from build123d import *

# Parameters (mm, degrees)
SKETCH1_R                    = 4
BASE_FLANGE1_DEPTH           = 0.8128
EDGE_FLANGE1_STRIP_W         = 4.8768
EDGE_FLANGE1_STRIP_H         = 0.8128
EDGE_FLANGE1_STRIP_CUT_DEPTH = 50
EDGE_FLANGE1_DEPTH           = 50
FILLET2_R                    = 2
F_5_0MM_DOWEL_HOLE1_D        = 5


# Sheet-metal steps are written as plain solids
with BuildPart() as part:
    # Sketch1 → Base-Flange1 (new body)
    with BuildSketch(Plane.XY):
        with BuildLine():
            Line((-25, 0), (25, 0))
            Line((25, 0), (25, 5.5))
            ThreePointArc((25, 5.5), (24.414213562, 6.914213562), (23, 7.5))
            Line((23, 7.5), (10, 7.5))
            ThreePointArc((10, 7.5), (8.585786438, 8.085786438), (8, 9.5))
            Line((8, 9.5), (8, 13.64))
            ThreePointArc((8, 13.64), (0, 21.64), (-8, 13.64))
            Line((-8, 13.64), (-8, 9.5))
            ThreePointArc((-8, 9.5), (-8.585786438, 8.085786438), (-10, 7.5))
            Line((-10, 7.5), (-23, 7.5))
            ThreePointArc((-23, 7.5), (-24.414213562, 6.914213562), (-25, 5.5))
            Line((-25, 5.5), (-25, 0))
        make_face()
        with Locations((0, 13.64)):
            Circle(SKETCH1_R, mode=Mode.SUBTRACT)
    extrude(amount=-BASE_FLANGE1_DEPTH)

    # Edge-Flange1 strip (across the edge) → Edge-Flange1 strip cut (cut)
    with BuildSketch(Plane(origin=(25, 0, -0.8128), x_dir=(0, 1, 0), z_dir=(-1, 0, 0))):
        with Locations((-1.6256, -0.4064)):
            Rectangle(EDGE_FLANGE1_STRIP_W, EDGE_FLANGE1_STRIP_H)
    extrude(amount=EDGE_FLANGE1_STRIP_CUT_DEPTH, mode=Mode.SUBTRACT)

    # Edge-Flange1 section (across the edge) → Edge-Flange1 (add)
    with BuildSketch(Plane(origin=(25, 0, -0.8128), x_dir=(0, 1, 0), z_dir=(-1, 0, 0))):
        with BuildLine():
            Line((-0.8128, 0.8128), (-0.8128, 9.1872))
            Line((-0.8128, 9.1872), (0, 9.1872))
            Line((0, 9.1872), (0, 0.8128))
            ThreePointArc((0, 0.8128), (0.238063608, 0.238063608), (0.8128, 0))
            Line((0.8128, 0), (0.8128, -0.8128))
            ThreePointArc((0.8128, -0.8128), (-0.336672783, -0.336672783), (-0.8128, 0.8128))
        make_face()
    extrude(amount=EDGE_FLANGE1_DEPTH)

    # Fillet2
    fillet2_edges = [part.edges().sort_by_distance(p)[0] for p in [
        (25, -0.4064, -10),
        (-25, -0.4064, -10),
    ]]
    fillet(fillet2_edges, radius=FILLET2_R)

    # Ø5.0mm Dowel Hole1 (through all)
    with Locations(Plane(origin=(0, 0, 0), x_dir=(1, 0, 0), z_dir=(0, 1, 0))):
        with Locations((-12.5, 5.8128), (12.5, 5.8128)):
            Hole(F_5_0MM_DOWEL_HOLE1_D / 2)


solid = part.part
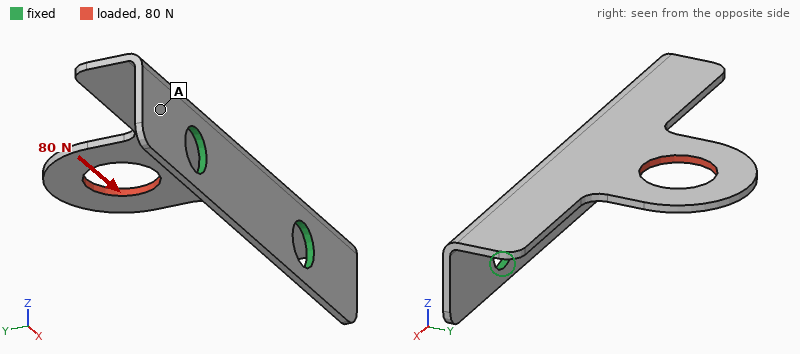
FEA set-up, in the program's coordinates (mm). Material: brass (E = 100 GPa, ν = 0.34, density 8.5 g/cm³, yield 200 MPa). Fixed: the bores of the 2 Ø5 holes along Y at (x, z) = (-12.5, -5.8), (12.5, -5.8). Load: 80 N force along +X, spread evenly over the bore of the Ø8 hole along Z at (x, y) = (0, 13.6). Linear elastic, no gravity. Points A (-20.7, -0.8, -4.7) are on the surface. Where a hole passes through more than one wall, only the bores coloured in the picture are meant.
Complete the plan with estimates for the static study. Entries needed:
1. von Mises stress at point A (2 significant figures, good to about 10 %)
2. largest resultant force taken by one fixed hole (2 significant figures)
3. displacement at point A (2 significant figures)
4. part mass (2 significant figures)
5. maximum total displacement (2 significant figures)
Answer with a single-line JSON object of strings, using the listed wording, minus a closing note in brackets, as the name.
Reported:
{"von Mises stress at point A": "12 MPa", "largest resultant force taken by one fixed hole": "59 N", "displacement at point A": "4.6 µm", "part mass": "6.6 g", "maximum total displacement": "30 µm"}
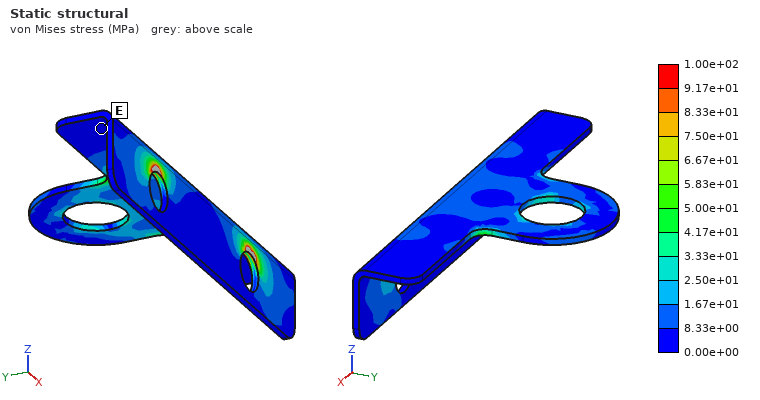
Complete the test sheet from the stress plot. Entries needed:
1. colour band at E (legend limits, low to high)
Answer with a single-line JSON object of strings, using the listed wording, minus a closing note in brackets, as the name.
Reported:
{"colour band at E": "0.00e+00 to 8.33e+00 MPa"}
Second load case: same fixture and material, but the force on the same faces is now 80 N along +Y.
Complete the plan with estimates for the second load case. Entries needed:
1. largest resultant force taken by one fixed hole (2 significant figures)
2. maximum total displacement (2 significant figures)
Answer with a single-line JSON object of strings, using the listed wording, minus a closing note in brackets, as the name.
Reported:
{"largest resultant force taken by one fixed hole": "45 N", "maximum total displacement": "70 µm"}
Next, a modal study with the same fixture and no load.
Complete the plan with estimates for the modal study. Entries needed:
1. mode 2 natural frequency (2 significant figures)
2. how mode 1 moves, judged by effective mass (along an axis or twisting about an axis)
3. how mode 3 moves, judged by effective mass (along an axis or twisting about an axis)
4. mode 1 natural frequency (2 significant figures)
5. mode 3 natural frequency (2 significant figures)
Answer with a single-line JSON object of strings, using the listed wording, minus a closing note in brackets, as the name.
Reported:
{"mode 2 natural frequency": "3400 Hz", "how mode 1 moves, judged by effective mass": "along Z", "how mode 3 moves, judged by effective mass": "along Z", "mode 1 natural frequency": "1200 Hz", "mode 3 natural frequency": "4300 Hz"}
